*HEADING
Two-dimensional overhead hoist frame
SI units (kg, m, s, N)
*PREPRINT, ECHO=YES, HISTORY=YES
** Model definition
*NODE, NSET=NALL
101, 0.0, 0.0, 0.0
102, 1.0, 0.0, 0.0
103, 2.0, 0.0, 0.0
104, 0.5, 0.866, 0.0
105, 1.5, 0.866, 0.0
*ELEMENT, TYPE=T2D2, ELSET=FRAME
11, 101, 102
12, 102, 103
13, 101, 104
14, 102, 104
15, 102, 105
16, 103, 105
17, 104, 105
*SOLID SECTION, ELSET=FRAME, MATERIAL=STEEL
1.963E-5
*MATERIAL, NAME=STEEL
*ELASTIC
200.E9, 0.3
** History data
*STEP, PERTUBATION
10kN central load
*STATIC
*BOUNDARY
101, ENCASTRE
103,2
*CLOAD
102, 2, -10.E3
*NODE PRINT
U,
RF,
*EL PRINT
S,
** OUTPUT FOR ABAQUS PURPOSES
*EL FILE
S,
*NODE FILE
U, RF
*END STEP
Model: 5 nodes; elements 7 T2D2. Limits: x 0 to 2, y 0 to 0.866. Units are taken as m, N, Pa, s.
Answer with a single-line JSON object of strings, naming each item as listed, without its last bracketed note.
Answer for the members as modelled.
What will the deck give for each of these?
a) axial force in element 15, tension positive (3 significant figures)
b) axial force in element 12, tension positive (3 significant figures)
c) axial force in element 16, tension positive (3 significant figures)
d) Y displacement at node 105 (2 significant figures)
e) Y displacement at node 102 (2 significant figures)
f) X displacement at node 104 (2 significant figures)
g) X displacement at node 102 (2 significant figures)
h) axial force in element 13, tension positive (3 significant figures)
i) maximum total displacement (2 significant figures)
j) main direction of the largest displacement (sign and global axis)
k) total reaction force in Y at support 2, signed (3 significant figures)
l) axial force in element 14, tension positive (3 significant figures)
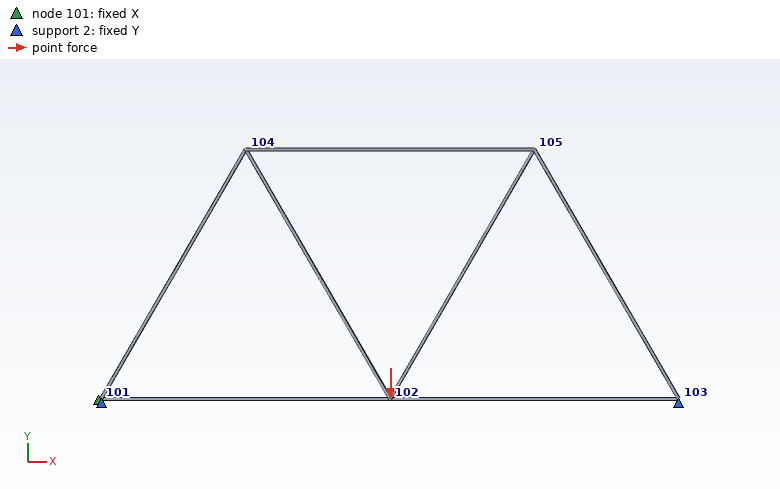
{"axial force in element 15, tension positive": "5770 N", "axial force in element 12, tension positive": "2890 N", "axial force in element 16, tension positive": "-5770 N", "Y displacement at node 105": "-0.0025 m", "Y displacement at node 102": "-0.0047 m", "X displacement at node 104": "0.0015 m", "X displacement at node 102": "7.4e-04 m", "axial force in element 13, tension positive": "-5770 N", "maximum total displacement": "0.0047 m", "main direction of the largest displacement": "-Y", "total reaction force in Y at support 2, signed": "10000 N", "axial force in element 14, tension positive": "5770 N"}
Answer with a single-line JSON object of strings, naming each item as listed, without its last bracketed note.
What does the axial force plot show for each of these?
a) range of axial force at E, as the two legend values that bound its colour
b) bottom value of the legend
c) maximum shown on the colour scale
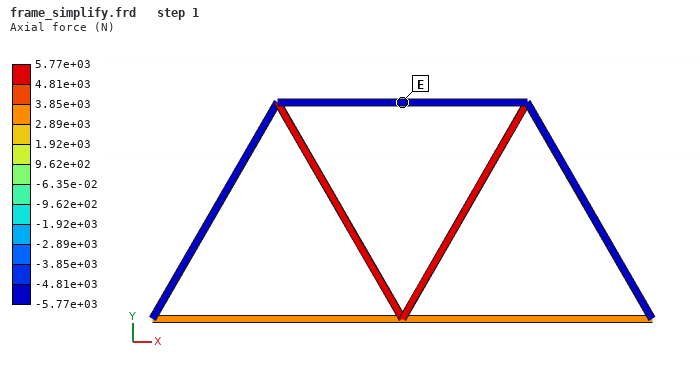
{"range of axial force at E, as the two legend values that bound its colour": "-5.77e+03 to -4.81e+03 N", "bottom value of the legend": "-5.77e+03 N", "maximum shown on the colour scale": "5.77e+03 N"}
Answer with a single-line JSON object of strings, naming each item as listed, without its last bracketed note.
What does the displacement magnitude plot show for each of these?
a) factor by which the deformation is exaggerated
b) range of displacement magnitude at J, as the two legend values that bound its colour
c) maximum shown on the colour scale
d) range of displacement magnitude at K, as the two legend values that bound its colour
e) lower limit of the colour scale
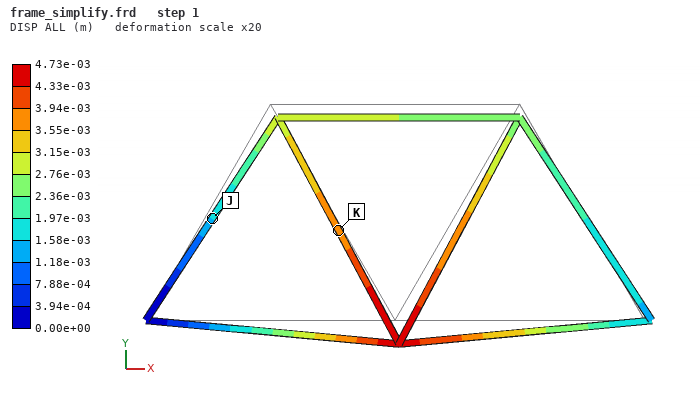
{"factor by which the deformation is exaggerated": "20", "range of displacement magnitude at J, as the two legend values that bound its colour": "1.18e-03 to 1.58e-03 m", "maximum shown on the colour scale": "4.73e-03 m", "range of displacement magnitude at K, as the two legend values that bound its colour": "3.55e-03 to 3.94e-03 m", "lower limit of the colour scale": "0.00e+00 m"}
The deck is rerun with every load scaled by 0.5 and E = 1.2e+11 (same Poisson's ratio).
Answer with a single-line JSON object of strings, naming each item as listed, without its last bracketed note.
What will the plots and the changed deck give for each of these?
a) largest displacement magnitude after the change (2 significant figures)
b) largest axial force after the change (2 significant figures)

{"largest displacement magnitude after the change": "0.0039 m", "largest axial force after the change": "2900 N"}
